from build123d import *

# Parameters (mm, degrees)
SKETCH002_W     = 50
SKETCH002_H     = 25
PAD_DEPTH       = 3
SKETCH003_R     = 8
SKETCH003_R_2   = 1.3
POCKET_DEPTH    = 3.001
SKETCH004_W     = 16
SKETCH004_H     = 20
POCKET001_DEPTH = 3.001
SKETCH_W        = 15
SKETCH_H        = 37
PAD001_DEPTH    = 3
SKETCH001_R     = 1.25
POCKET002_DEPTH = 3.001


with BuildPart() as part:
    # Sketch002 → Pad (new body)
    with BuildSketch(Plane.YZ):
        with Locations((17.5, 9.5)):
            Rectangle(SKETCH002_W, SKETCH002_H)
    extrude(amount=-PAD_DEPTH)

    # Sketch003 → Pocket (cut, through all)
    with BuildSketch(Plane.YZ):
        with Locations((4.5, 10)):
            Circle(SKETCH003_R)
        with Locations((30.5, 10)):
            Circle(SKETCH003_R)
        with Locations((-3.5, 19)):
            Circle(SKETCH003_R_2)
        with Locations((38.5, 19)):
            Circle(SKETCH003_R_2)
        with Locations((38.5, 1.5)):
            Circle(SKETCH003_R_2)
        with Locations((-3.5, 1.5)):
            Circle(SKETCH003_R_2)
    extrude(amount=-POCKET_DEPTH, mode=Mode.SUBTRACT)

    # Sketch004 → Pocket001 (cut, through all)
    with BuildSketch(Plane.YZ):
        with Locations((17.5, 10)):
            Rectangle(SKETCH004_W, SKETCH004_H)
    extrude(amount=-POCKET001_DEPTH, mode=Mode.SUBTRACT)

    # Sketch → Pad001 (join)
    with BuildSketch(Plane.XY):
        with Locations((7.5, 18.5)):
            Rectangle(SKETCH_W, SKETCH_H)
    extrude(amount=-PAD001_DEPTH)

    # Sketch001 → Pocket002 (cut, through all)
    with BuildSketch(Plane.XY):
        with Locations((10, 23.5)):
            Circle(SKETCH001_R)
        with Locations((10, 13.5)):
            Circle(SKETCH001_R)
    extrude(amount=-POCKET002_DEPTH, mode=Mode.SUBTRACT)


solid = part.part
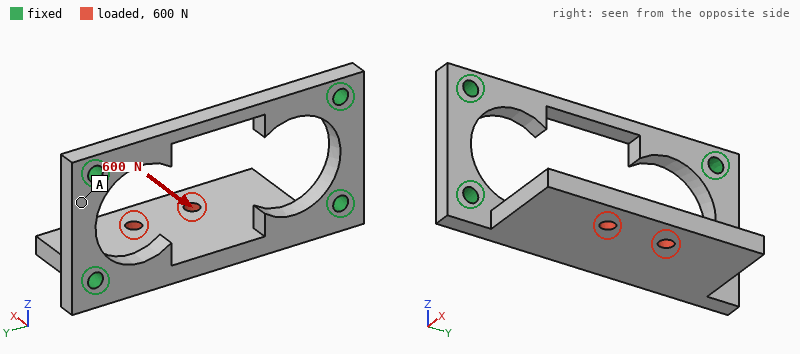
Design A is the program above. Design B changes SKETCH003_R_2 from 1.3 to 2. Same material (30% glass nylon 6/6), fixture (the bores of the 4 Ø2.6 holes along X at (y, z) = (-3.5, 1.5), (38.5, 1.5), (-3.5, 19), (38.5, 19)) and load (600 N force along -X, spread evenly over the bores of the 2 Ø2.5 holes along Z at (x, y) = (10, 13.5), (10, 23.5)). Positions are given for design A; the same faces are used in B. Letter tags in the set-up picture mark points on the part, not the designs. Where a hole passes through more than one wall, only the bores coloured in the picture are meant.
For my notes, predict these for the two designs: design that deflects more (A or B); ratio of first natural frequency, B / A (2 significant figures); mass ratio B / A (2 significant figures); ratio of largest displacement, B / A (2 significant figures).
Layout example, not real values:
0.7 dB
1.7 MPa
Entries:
A
1.1
0.97
0.76
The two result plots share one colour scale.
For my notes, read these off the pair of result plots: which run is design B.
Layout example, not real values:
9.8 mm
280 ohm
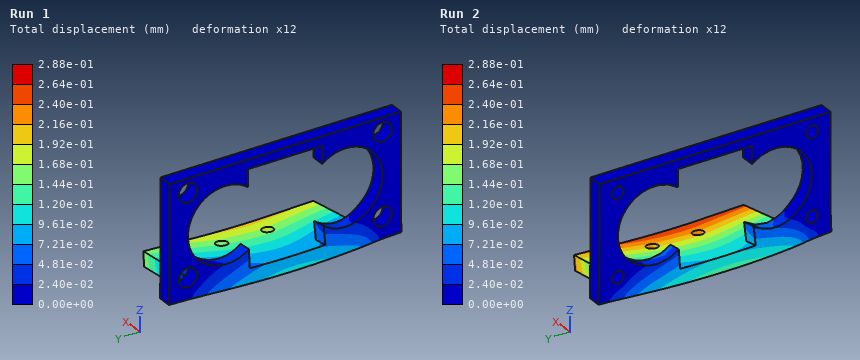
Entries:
Run 1
